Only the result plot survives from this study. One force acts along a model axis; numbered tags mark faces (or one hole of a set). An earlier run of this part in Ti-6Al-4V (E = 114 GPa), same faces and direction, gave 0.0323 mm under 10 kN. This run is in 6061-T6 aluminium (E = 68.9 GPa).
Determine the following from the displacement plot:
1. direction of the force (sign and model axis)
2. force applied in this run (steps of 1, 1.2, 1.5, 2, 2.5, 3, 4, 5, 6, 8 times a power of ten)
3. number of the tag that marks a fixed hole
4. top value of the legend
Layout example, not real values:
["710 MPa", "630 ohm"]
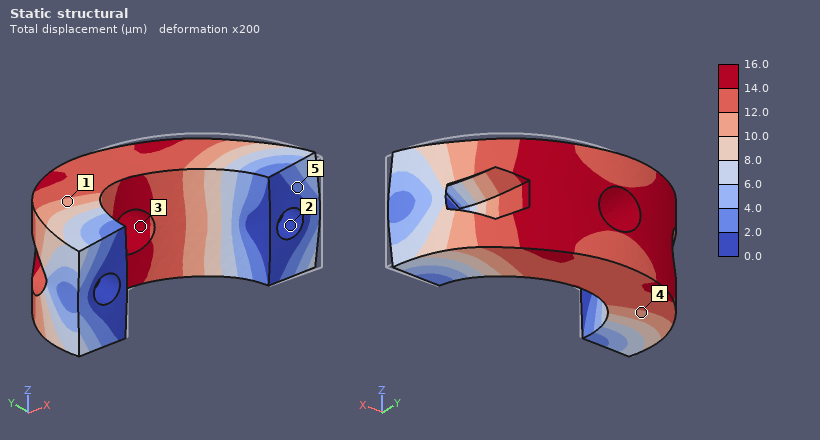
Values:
["-X", "3 kN", "2", "16.0 µm"]
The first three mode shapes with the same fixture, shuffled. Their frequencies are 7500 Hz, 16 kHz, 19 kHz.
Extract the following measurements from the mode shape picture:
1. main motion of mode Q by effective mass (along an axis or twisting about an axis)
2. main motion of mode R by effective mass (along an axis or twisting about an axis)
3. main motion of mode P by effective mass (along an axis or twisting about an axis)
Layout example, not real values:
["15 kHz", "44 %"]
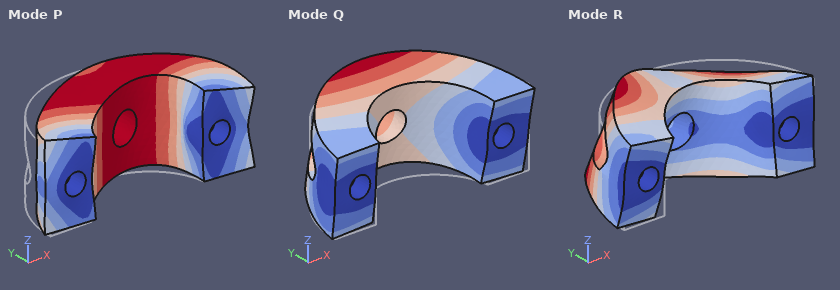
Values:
["along Z", "twisting about Y", "along X"]
